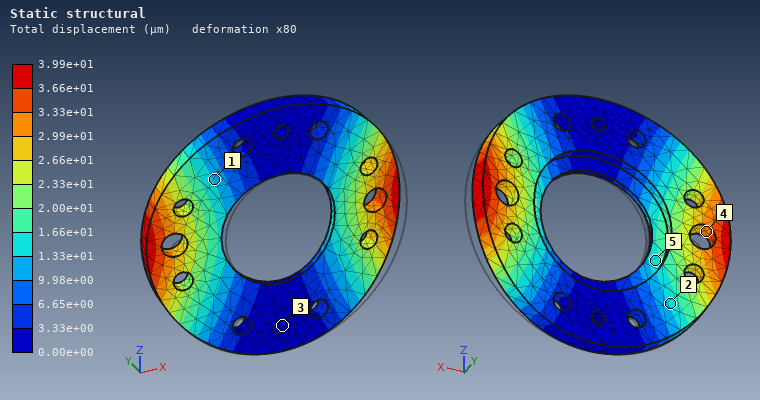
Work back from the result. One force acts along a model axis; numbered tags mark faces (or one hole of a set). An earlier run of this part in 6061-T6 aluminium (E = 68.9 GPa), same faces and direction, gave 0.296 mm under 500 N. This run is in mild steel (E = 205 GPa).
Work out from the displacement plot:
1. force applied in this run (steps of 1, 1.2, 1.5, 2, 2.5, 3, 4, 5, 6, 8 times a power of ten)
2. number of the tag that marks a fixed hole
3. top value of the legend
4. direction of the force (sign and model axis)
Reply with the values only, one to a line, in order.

200 N
3
3.99e+01 µm
+Y
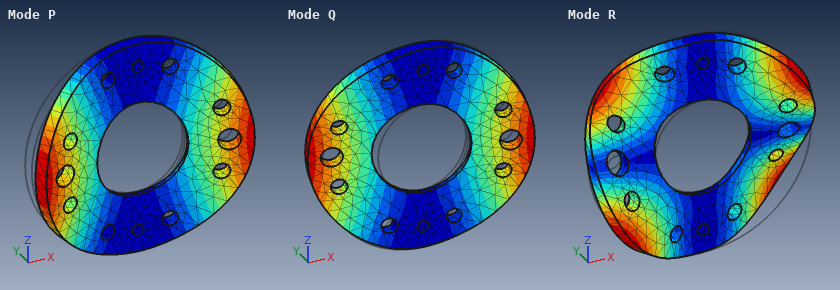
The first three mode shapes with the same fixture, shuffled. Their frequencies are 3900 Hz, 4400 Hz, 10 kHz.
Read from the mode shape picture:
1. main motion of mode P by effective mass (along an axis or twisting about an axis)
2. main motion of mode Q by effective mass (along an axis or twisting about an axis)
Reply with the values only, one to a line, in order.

along Y
twisting about Z
